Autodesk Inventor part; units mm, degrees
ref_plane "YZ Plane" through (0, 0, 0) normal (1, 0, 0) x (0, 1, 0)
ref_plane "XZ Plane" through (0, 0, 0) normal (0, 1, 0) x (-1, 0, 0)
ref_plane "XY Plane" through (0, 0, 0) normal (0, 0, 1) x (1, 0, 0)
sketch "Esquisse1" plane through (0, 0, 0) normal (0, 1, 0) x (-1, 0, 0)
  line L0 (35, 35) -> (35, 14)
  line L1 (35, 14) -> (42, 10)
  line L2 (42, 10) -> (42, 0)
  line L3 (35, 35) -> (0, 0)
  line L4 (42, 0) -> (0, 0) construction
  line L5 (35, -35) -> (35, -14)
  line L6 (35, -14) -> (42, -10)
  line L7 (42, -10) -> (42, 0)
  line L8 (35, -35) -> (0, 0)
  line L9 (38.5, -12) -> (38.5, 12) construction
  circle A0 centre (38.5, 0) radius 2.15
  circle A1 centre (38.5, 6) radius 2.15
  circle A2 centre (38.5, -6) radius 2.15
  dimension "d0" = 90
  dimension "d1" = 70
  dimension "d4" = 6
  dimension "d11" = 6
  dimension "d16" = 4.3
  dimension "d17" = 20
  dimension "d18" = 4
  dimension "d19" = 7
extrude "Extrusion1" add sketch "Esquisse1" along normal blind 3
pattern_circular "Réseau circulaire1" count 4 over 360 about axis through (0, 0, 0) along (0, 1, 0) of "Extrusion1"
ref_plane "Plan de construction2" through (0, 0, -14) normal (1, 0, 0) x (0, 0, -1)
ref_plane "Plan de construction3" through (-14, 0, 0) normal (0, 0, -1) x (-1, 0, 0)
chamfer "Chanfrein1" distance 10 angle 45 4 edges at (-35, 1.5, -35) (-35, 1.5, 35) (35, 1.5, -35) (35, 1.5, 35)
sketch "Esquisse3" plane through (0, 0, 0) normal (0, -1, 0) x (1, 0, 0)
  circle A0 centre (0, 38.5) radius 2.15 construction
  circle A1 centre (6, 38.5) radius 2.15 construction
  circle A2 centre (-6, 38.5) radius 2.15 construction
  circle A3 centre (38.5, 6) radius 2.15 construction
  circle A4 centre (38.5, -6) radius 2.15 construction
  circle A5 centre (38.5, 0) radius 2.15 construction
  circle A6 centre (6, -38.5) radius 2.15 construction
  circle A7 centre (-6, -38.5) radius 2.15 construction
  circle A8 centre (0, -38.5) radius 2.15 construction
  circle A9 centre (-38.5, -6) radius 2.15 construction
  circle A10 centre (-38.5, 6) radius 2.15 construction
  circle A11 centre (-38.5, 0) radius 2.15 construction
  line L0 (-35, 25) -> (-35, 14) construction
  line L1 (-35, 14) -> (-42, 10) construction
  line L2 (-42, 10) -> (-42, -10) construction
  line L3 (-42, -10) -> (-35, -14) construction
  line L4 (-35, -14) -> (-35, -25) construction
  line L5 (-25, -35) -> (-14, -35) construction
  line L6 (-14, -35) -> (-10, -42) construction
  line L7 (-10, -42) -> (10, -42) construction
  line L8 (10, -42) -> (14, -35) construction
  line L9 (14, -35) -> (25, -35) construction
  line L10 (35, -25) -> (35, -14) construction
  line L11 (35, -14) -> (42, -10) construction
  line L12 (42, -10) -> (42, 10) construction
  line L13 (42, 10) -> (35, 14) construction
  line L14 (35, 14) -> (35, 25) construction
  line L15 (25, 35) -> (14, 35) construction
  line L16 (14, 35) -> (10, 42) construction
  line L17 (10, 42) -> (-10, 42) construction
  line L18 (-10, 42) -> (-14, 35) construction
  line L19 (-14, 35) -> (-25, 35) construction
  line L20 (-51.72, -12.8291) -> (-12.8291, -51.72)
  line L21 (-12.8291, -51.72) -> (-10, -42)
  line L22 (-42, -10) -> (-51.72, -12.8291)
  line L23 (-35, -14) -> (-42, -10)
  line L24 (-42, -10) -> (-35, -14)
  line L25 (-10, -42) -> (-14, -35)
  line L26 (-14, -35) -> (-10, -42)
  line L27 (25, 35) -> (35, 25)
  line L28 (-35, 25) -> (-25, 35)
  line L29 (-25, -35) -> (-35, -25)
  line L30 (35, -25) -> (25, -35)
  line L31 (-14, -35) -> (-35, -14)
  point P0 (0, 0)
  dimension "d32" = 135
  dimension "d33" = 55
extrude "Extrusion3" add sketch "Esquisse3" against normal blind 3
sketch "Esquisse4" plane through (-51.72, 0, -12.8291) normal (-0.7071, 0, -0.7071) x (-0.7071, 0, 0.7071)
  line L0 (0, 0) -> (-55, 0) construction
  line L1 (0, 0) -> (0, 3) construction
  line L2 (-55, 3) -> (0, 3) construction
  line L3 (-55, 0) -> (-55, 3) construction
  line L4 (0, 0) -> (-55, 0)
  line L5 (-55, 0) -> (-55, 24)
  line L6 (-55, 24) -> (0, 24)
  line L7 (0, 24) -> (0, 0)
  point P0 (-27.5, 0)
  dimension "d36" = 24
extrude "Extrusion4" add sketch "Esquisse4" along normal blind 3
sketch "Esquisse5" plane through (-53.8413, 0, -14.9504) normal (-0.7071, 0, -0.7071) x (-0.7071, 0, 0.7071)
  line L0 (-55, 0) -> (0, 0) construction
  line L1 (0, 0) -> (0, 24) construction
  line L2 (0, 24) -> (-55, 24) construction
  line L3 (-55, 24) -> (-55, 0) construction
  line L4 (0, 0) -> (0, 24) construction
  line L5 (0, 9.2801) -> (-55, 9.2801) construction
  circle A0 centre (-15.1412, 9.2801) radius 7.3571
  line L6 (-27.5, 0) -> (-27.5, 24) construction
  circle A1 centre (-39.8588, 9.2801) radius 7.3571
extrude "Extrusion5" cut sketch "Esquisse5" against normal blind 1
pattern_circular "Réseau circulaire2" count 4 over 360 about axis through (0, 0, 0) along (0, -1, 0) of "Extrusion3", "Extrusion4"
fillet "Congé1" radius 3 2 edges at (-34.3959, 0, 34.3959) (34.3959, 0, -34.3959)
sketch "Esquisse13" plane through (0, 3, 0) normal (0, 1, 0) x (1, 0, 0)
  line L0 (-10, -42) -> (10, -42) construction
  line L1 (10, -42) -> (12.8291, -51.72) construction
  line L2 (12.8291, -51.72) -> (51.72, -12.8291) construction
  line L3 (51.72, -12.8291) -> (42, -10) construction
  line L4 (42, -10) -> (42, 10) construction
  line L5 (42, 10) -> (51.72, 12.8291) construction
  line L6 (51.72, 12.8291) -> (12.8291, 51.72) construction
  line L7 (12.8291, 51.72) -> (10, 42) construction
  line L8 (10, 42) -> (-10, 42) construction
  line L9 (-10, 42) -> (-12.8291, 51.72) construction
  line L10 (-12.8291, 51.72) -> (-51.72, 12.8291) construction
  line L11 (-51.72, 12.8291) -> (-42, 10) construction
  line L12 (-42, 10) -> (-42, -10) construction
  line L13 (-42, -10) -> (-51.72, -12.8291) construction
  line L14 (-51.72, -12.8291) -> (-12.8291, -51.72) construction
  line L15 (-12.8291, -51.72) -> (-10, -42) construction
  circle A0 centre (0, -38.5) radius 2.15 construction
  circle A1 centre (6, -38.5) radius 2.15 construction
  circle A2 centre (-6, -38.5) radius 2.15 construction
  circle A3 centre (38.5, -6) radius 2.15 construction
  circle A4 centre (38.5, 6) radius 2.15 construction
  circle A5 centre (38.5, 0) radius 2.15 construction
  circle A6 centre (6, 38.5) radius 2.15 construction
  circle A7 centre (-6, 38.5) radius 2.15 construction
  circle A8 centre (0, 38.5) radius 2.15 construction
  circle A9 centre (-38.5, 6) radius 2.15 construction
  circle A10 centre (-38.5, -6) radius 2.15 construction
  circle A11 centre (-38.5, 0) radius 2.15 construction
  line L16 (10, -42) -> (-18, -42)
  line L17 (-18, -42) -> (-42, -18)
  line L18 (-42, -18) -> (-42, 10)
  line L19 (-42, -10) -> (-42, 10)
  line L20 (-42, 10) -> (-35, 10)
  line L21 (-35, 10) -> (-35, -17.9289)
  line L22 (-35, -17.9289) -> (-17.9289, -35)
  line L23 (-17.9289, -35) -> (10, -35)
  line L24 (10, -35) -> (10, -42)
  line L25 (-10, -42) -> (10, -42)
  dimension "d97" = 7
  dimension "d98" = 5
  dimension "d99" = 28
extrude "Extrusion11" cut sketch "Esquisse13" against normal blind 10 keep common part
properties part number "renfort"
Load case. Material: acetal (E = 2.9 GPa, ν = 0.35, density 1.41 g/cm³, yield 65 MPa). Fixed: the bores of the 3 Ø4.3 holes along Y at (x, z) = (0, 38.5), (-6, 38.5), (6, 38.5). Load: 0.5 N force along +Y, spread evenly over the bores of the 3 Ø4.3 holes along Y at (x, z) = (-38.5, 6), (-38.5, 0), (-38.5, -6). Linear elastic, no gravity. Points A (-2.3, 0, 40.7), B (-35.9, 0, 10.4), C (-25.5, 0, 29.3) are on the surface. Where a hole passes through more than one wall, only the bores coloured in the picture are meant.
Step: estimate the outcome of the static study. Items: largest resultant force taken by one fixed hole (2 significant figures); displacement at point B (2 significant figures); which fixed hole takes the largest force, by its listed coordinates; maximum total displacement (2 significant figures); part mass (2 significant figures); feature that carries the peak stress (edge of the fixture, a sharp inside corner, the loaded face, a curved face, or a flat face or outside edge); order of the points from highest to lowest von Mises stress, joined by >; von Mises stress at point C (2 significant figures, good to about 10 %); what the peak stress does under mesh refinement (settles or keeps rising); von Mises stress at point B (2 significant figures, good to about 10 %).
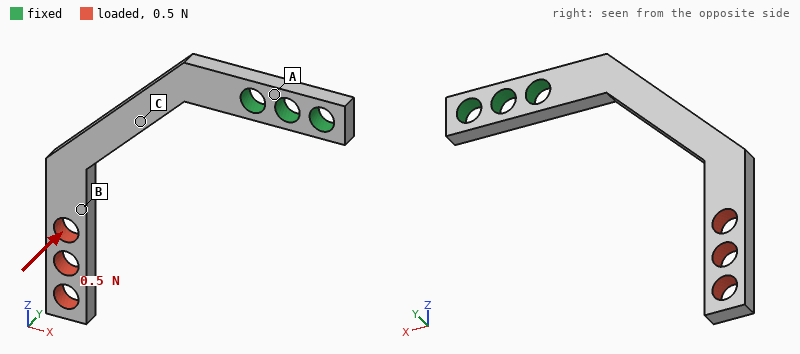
0.55 N
0.46 mm
(-6, 38.5)
0.88 mm
1.9 g
a sharp inside corner
C > B > A
2.2 MPa
keeps rising
0.55 MPa
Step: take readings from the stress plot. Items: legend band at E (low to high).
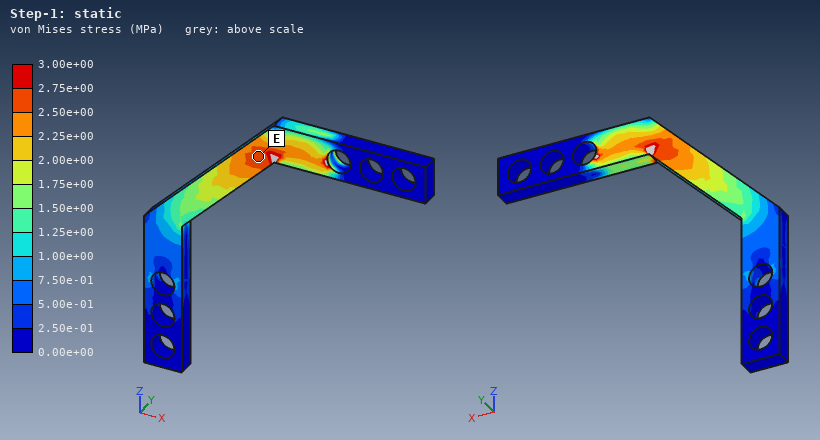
2.50e+00 to 2.75e+00 MPa
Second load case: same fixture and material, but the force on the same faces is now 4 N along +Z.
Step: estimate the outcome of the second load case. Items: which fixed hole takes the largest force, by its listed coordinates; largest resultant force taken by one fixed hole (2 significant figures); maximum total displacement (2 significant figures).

(-6, 38.5)
5.7 N
0.85 mm
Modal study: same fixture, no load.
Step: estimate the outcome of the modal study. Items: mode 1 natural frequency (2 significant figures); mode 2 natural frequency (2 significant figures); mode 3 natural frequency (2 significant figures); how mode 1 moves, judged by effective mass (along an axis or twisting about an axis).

180 Hz
330 Hz
750 Hz
along Y
